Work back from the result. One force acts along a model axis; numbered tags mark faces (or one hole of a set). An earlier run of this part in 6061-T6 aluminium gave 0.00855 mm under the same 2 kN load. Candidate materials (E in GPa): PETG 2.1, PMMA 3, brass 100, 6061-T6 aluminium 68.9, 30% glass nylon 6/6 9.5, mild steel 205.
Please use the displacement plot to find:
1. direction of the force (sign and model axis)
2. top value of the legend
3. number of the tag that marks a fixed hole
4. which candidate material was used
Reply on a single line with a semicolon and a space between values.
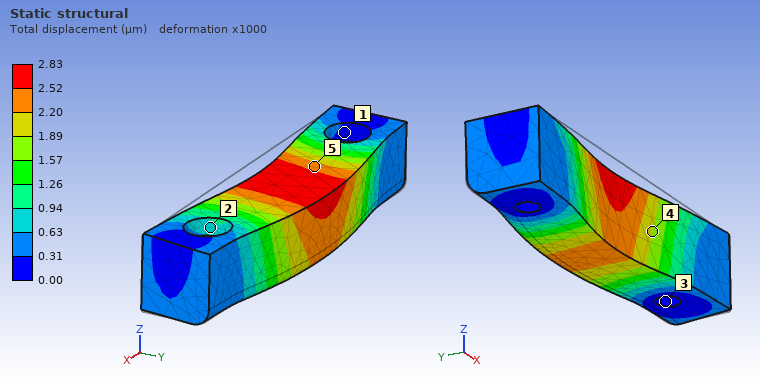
+Y; 2.83 µm; 3; mild steel
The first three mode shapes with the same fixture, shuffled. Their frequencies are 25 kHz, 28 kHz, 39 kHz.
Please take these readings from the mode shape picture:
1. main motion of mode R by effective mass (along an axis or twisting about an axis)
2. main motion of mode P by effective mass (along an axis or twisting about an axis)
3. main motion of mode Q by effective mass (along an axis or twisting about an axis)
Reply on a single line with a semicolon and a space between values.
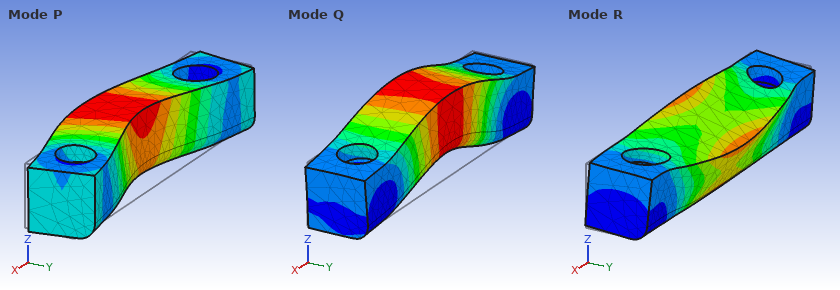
twisting about X; along Y; along Z
